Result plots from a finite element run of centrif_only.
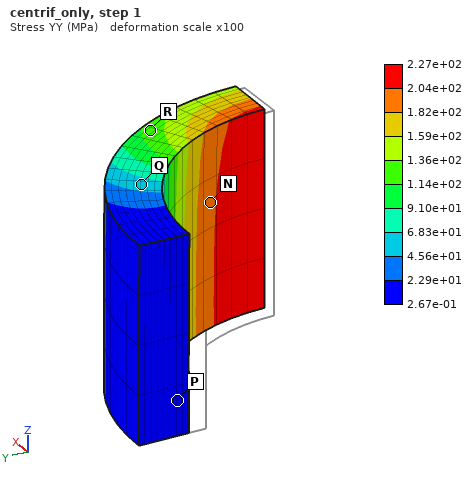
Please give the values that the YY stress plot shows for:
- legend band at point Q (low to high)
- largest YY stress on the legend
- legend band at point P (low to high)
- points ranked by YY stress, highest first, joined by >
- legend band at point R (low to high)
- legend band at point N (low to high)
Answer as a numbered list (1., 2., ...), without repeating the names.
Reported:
1. 4.56e+01 to 6.83e+01 MPa
2. 2.27e+02 MPa
3. 2.67e-01 to 2.29e+01 MPa
4. N > R > Q > P
5. 1.14e+02 to 1.36e+02 MPa
6. 1.82e+02 to 2.04e+02 MPa
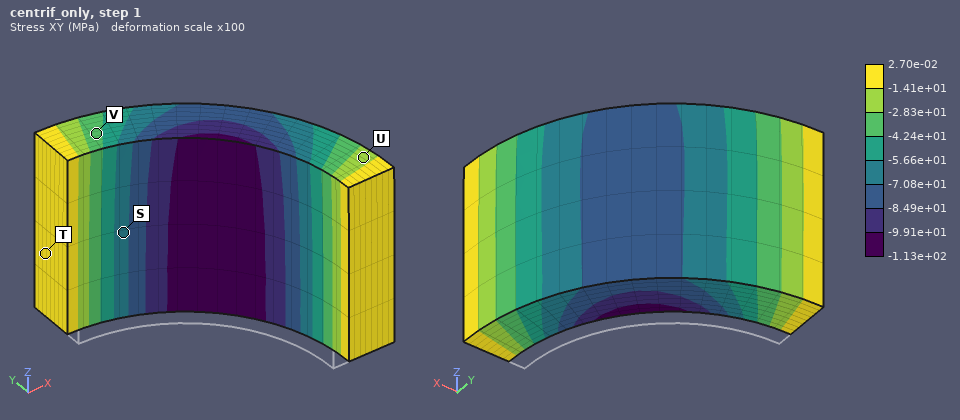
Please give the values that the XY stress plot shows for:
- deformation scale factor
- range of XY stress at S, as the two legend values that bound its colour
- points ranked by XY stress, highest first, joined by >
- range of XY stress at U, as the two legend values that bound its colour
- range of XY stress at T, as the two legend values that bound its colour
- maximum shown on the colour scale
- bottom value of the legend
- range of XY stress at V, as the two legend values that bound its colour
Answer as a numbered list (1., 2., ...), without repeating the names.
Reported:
1. 100
2. -7.08e+01 to -5.66e+01 MPa
3. T > U > V > S
4. -2.83e+01 to -1.41e+01 MPa
5. -1.41e+01 to 2.70e-02 MPa
6. 2.70e-02 MPa
7. -1.13e+02 MPa
8. -4.24e+01 to -2.83e+01 MPa
